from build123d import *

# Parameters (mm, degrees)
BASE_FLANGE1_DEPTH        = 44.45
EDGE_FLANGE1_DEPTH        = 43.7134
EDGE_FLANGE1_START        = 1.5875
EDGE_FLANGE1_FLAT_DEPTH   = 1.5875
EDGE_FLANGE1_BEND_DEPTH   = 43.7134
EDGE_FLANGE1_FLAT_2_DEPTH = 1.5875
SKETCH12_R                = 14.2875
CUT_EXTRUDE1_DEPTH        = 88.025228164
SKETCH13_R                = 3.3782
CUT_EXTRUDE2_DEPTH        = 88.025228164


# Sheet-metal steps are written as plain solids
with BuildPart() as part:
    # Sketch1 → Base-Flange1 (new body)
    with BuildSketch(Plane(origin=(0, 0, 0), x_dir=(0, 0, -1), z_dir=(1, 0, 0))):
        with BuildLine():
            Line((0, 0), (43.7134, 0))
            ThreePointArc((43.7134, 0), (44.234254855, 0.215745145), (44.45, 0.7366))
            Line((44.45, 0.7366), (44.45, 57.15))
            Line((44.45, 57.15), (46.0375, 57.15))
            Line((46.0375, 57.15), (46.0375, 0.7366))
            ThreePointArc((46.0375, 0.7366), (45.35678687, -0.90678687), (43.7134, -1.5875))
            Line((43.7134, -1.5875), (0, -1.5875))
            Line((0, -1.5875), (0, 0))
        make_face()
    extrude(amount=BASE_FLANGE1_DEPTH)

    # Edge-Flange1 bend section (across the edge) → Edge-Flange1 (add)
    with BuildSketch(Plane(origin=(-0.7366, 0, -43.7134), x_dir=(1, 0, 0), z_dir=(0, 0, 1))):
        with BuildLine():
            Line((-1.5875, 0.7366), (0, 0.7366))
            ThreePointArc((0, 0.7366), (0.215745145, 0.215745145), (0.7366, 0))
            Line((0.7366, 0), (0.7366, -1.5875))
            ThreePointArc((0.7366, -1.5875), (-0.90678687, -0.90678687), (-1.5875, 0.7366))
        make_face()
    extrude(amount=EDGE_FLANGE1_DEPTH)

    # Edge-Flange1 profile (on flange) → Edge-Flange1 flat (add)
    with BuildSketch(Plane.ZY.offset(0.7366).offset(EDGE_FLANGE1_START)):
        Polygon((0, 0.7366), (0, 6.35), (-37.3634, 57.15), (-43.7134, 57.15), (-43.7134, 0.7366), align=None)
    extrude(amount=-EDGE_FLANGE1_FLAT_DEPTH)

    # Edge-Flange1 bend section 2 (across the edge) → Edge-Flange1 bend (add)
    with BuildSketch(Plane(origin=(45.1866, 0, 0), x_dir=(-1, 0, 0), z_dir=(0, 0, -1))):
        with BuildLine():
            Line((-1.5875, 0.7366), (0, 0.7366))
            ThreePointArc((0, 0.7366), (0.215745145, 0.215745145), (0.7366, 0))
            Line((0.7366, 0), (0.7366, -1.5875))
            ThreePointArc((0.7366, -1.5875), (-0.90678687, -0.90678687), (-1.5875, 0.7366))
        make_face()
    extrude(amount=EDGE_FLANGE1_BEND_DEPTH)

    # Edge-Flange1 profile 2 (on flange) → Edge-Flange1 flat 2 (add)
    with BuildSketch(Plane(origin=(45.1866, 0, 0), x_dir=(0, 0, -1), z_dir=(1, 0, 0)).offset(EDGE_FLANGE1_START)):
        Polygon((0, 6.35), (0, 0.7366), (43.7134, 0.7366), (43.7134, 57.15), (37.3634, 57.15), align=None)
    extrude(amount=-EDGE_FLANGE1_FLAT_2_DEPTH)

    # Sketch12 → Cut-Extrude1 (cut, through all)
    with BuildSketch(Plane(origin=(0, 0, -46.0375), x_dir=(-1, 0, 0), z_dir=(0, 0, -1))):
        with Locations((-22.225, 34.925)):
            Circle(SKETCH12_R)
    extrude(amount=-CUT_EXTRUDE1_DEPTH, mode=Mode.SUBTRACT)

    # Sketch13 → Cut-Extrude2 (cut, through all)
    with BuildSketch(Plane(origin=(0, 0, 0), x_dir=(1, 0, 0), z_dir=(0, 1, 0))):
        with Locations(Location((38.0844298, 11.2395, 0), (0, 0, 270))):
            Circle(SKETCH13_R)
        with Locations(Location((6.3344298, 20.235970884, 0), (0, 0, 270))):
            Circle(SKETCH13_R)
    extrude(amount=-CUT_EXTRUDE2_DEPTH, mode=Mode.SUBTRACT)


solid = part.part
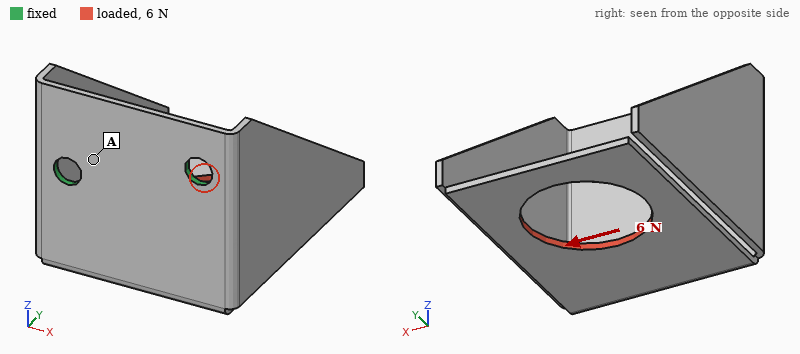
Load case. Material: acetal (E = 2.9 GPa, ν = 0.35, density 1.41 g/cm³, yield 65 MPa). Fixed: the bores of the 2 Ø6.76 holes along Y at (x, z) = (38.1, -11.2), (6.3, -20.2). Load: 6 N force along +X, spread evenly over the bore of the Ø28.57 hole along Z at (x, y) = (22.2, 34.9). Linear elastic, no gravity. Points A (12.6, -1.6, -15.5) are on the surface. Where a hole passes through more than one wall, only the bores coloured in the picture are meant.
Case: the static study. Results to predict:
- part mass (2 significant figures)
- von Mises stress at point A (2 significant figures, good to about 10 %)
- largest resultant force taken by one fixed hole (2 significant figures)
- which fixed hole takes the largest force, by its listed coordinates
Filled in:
16 g
1.3 MPa
8.5 N
(6.3, -20.2)
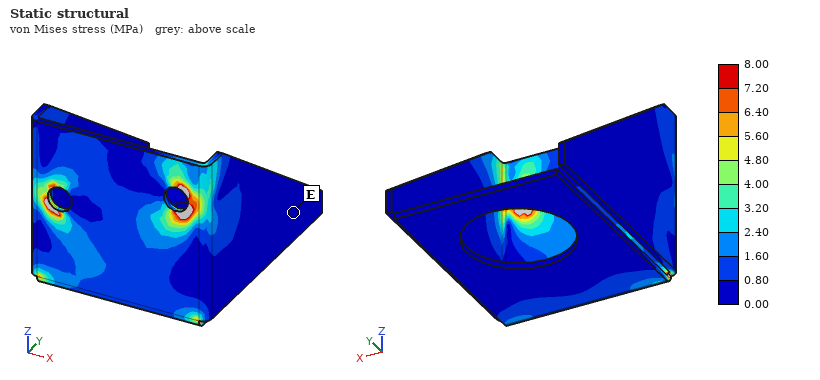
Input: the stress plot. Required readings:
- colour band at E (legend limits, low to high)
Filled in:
0.00 to 0.80 MPa
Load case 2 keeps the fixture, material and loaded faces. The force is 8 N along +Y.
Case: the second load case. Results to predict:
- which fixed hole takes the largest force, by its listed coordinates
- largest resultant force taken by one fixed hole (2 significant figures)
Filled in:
(6.3, -20.2)
4.6 N
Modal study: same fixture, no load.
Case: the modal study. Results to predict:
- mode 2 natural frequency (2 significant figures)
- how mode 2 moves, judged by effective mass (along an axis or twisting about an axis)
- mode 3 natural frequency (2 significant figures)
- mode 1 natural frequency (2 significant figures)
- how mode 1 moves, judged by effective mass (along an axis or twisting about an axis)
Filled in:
140 Hz
along X
150 Hz
96 Hz
along Z
